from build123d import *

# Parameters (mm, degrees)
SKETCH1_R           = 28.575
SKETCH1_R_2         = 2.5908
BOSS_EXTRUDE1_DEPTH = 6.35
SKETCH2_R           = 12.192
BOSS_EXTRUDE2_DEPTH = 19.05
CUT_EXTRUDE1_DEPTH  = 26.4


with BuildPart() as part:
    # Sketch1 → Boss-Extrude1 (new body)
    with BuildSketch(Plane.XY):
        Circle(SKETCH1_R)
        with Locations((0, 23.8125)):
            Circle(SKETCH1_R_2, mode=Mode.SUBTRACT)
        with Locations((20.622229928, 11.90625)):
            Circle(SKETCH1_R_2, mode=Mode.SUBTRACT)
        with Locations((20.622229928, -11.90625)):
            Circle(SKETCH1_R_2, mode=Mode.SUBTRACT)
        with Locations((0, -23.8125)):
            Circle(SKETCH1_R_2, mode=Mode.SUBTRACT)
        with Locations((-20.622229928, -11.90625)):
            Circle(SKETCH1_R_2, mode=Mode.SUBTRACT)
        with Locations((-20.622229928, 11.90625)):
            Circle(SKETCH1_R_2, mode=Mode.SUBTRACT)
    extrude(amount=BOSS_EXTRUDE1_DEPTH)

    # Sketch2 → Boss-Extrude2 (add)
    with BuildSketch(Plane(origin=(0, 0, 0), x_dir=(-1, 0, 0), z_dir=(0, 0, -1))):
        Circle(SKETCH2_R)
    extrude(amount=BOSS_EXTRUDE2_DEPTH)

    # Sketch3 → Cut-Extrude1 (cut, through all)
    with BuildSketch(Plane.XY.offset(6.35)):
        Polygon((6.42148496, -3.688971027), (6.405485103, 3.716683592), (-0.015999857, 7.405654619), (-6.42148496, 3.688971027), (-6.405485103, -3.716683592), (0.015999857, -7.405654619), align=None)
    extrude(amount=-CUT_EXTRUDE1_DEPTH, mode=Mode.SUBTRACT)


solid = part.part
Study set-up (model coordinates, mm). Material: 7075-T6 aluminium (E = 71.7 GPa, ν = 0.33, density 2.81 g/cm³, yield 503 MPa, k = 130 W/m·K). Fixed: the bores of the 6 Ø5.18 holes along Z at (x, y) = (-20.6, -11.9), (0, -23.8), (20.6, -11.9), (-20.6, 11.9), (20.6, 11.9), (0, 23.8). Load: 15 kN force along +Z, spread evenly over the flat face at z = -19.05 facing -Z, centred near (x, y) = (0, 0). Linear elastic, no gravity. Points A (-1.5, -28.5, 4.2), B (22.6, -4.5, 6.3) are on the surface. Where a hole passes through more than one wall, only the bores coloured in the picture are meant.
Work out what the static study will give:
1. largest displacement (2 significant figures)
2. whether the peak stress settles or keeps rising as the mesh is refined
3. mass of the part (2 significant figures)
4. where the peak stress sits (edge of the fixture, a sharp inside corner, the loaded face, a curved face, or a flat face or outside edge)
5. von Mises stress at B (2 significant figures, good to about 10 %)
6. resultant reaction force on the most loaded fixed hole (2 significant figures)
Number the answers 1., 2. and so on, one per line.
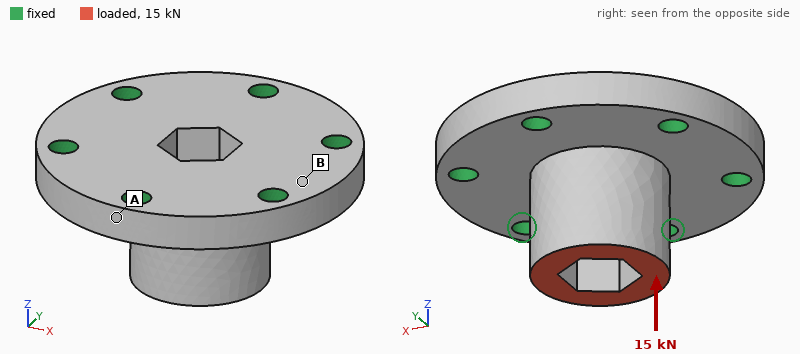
1. 51 µm
2. keeps rising
3. 58 g
4. edge of the fixture
5. 45 MPa
6. 2.7 kN
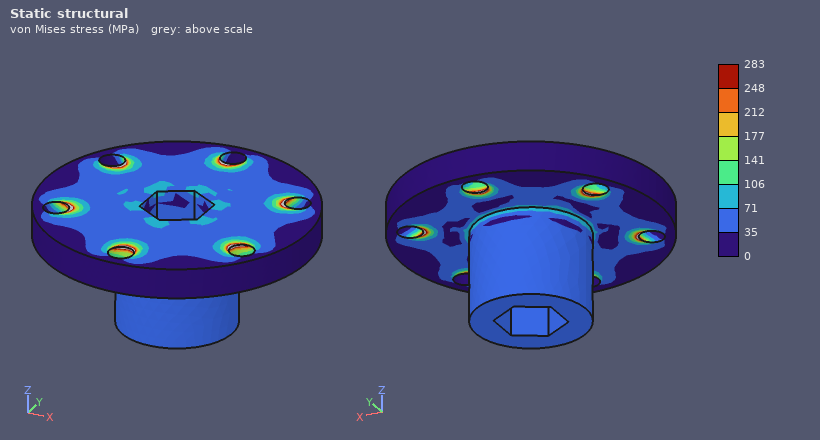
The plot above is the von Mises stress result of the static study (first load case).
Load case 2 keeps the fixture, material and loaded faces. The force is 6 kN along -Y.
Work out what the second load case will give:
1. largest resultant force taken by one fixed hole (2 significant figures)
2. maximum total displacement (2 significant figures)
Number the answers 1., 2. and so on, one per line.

1. 2.9 kN
2. 96 µm
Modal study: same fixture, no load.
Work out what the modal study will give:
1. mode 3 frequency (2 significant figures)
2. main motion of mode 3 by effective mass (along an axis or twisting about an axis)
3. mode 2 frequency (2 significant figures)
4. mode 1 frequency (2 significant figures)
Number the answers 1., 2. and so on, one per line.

1. 18 kHz
2. along Z
3. 16 kHz
4. 16 kHz
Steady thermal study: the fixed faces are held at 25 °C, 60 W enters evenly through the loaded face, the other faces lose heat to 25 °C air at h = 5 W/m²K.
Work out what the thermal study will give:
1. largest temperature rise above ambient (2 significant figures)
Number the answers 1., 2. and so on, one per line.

1. 39 K
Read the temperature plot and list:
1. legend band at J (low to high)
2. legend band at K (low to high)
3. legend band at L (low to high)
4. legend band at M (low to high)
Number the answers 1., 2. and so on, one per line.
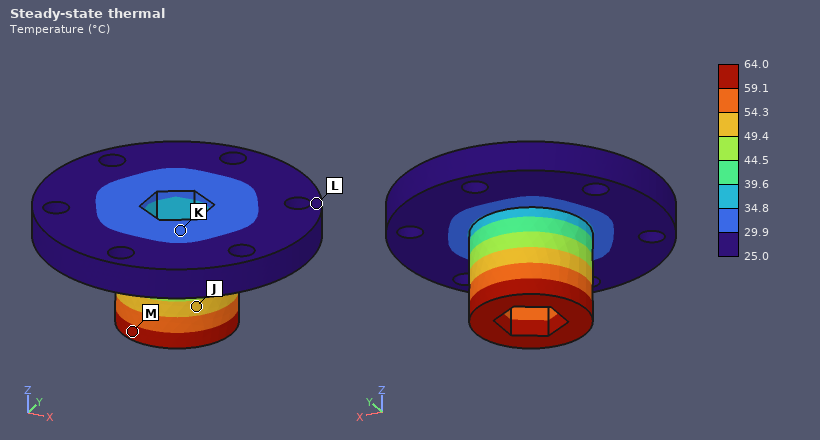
1. 49.4 to 54.3 °C
2. 29.9 to 34.8 °C
3. 25.0 to 29.9 °C
4. 59.1 to 64.0 °C
